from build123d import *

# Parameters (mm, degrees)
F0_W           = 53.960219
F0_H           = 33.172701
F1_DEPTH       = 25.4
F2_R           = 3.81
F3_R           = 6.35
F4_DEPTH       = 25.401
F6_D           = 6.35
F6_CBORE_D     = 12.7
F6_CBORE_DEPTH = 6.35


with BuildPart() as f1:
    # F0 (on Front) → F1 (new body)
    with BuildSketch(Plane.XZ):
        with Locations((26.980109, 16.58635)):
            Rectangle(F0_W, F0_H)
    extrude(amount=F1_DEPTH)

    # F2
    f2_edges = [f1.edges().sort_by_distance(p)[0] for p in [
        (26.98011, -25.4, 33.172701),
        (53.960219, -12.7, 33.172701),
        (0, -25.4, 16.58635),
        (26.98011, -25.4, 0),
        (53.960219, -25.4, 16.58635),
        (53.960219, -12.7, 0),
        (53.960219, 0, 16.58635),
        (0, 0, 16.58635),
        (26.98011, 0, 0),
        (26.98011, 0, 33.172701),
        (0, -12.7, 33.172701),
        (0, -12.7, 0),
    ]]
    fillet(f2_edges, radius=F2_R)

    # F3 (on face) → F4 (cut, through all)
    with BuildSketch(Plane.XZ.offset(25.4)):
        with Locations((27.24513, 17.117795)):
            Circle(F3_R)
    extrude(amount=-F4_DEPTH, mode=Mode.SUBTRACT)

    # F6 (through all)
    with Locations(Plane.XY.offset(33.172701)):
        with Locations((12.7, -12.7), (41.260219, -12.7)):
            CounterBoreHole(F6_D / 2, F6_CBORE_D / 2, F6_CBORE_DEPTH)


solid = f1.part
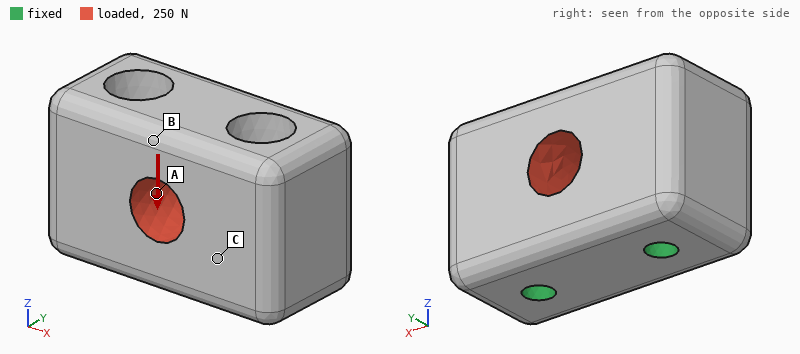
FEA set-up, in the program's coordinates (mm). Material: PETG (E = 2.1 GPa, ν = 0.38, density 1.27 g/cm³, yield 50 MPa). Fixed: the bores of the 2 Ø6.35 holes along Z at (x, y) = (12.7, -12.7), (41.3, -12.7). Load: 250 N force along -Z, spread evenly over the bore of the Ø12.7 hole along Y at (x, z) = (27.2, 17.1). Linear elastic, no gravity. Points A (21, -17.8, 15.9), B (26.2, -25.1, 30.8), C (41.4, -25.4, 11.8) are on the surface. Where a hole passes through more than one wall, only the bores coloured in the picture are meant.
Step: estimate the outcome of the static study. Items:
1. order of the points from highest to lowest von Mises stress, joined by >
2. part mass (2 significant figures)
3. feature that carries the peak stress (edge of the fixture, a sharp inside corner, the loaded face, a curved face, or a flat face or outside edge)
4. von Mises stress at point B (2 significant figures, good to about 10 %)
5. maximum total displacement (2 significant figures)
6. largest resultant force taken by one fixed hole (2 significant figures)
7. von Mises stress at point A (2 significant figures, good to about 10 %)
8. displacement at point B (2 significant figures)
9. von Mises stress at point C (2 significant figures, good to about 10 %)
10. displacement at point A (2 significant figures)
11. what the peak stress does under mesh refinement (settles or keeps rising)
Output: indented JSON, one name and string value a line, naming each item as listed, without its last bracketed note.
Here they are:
{
  "order of the points from highest to lowest von Mises stress, joined by >": "A > B > C",
  "part mass": "48 g",
  "feature that carries the peak stress": "edge of the fixture",
  "von Mises stress at point B": "0.29 MPa",
  "maximum total displacement": "4.2 µm",
  "largest resultant force taken by one fixed hole": "130 N",
  "von Mises stress at point A": "0.47 MPa",
  "displacement at point B": "3.6 µm",
  "von Mises stress at point C": "0.14 MPa",
  "displacement at point A": "2.4 µm",
  "what the peak stress does under mesh refinement": "keeps rising"
}
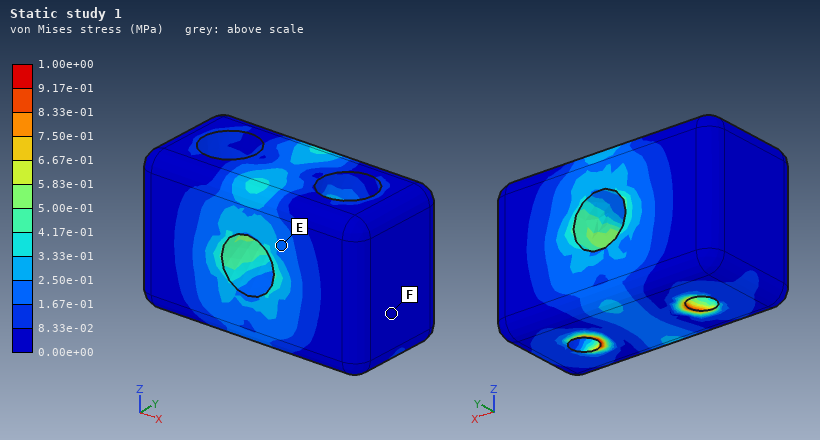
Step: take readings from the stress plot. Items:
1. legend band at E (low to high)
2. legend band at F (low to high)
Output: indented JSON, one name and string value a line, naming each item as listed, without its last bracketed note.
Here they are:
{
  "legend band at E": "1.67e-01 to 2.50e-01 MPa",
  "legend band at F": "0.00e+00 to 8.33e-02 MPa"
}
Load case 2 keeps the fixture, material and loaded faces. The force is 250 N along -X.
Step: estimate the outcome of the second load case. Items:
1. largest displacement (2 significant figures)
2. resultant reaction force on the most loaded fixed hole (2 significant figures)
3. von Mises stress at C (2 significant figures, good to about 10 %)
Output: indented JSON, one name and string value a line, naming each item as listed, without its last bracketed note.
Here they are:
{
  "largest displacement": "2.3 µm",
  "resultant reaction force on the most loaded fixed hole": "130 N",
  "von Mises stress at C": "0.14 MPa"
}
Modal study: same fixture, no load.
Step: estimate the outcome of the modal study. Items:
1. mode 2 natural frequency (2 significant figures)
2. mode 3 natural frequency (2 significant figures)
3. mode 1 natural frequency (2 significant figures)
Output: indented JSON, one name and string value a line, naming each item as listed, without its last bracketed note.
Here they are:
{
  "mode 2 natural frequency": "8200 Hz",
  "mode 3 natural frequency": "8500 Hz",
  "mode 1 natural frequency": "7900 Hz"
}
